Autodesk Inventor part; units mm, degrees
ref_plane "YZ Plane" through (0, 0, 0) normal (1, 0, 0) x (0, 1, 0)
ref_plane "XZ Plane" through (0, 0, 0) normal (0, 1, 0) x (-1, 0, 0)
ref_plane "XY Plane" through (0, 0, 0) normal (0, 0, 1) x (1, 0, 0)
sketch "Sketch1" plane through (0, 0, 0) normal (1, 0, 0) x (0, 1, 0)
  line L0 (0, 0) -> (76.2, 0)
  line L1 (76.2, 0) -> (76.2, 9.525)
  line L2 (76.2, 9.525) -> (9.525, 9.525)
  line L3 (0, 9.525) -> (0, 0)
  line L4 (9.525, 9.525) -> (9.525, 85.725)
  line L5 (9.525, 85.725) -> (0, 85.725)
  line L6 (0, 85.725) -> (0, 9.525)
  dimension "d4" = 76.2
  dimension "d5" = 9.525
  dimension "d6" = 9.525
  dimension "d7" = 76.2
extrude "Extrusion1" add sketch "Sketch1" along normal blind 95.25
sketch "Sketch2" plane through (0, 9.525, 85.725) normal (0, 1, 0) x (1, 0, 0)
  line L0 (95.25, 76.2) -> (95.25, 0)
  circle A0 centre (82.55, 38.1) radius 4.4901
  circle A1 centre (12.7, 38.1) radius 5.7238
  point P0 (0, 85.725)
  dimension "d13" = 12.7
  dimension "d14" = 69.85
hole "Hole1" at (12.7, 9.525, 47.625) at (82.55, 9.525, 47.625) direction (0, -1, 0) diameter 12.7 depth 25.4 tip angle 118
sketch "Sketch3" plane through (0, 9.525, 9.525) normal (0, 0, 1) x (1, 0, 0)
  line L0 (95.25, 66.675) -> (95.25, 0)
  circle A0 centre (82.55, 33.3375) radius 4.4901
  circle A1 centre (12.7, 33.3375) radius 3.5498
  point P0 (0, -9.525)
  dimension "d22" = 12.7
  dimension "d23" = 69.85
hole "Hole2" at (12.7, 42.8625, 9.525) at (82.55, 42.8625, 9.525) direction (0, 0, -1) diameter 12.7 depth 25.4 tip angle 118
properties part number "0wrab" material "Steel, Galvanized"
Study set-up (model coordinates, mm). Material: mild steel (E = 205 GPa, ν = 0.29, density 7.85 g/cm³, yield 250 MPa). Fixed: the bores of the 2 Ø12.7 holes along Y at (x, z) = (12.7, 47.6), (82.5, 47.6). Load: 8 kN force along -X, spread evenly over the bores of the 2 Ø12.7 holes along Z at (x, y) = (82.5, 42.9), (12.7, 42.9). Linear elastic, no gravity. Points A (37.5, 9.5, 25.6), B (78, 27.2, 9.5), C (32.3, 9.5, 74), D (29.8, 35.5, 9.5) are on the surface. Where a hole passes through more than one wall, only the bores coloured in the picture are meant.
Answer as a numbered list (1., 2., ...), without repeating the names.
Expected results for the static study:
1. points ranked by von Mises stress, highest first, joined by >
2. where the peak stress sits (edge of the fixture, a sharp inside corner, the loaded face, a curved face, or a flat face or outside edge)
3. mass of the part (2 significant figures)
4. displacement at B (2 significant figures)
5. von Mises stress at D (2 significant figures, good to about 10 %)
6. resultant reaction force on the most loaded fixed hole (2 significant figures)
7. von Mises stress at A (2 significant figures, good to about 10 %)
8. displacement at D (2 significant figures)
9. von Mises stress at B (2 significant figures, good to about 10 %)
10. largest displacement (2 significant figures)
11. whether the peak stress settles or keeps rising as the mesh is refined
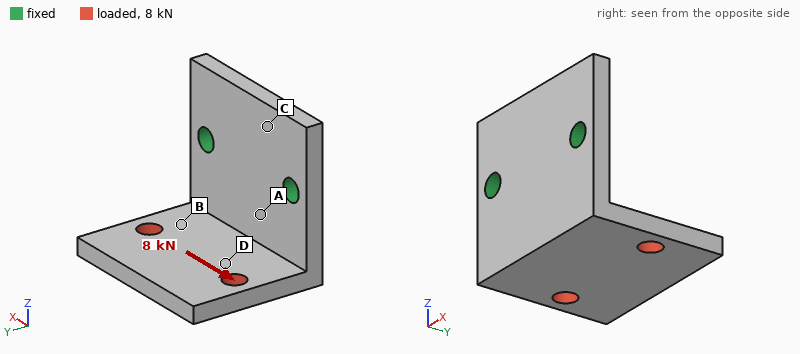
1. A > B > D > C
2. edge of the fixture
3. 1.0 kg
4. 0.080 mm
5. 38 MPa
6. 7.3 kN
7. 89 MPa
8. 0.080 mm
9. 57 MPa
10. 0.19 mm
11. keeps rising
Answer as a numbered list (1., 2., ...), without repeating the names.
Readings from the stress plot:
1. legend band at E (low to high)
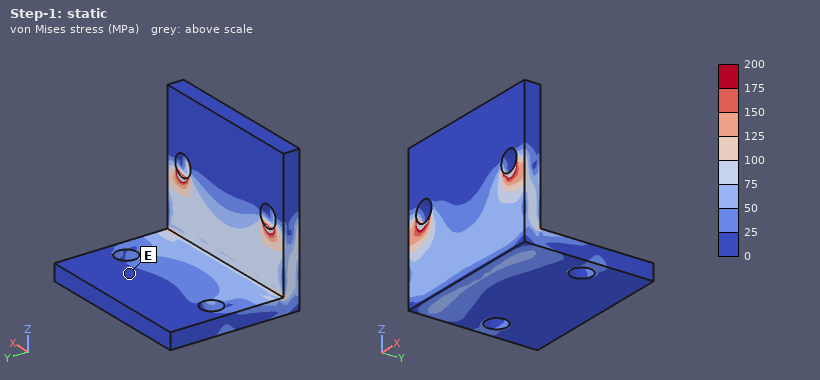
1. 0 to 25 MPa
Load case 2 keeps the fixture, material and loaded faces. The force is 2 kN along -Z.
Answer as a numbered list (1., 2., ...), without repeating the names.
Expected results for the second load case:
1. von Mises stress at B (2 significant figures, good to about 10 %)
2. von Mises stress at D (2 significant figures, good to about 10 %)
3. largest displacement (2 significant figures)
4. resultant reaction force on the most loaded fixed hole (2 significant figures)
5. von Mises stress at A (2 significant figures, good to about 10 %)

1. 20 MPa
2. 12 MPa
3. 0.21 mm
4. 1.0 kN
5. 46 MPa
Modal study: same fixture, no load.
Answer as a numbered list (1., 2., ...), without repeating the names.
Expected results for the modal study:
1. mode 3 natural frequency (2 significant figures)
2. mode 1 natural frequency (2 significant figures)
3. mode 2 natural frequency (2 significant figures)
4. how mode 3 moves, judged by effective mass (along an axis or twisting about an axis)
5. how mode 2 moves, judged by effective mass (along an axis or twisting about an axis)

1. 2400 Hz
2. 810 Hz
3. 1700 Hz
4. along Y
5. along X
